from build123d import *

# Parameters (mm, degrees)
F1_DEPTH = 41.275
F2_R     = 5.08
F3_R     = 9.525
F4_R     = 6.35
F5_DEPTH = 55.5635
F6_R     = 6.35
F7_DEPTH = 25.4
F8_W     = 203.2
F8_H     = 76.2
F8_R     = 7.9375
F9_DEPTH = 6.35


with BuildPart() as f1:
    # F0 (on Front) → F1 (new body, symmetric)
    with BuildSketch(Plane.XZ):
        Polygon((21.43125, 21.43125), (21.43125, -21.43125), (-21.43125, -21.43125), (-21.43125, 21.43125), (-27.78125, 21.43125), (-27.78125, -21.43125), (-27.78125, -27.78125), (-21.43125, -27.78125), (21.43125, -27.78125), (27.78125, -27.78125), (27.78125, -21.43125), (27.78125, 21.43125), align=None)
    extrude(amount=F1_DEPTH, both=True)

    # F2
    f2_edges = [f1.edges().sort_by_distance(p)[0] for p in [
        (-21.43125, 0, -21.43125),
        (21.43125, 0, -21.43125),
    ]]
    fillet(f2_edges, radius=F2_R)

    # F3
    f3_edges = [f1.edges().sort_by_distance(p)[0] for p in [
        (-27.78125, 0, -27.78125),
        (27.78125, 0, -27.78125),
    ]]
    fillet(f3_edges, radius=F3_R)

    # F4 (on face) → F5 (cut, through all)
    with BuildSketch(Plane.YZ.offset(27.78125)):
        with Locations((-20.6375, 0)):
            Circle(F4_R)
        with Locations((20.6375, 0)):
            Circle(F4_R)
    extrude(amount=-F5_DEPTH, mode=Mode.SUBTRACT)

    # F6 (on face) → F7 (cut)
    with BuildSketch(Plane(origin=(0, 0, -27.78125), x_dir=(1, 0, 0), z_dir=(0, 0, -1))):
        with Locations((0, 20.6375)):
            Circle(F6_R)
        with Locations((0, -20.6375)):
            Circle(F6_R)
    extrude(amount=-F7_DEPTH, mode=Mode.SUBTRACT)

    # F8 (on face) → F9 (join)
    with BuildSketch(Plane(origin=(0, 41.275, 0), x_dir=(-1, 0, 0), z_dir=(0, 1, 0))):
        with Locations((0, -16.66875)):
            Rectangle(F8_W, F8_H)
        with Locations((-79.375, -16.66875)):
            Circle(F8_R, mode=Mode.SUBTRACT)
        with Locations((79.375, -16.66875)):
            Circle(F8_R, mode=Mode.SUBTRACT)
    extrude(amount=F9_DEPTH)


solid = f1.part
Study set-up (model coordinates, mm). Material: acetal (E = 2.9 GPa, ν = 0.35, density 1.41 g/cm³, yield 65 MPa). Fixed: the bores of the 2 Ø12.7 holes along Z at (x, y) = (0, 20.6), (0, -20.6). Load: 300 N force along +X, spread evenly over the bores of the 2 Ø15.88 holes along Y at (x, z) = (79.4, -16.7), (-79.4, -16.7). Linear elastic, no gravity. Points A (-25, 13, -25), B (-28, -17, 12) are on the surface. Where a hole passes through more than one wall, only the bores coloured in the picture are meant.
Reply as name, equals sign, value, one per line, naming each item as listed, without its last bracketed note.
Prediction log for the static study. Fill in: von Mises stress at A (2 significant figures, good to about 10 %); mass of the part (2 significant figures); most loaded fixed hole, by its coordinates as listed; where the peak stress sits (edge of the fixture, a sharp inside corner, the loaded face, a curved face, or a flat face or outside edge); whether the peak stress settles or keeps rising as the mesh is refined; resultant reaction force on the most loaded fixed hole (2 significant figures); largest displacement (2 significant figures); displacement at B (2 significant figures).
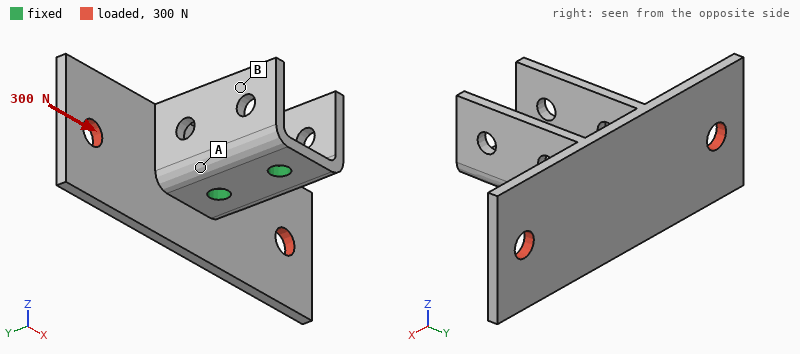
von Mises stress at A = 1.5 MPa
mass of the part = 230 g
most loaded fixed hole, by its coordinates as listed = (0, 20.6)
where the peak stress sits = edge of the fixture
whether the peak stress settles or keeps rising as the mesh is refined = keeps rising
resultant reaction force on the most loaded fixed hole = 400 N
largest displacement = 0.39 mm
displacement at B = 0.082 mm
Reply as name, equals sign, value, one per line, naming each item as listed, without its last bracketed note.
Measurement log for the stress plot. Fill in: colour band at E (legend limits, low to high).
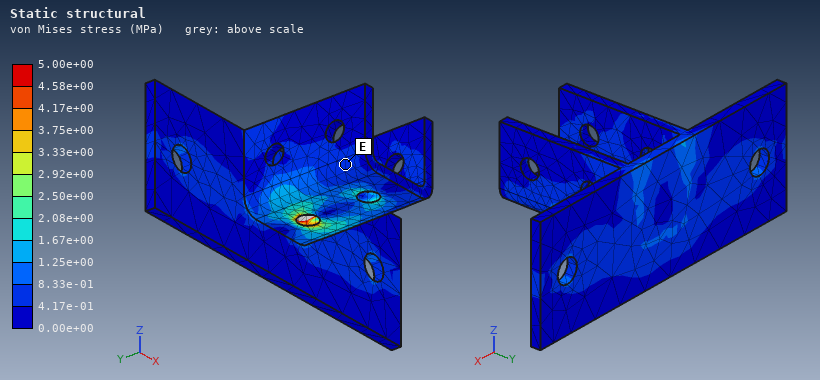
colour band at E = 4.17e-01 to 8.33e-01 MPa
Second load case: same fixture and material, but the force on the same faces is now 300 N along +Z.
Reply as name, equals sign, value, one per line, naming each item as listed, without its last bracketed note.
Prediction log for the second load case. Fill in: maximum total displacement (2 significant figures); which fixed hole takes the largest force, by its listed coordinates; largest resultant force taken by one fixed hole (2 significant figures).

maximum total displacement = 0.24 mm
which fixed hole takes the largest force, by its listed coordinates = (0, 20.6)
largest resultant force taken by one fixed hole = 390 N
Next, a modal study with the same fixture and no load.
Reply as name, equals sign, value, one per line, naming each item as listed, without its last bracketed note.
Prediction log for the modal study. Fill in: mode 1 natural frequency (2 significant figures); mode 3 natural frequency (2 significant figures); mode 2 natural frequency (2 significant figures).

mode 1 natural frequency = 180 Hz
mode 3 natural frequency = 230 Hz
mode 2 natural frequency = 230 Hz
